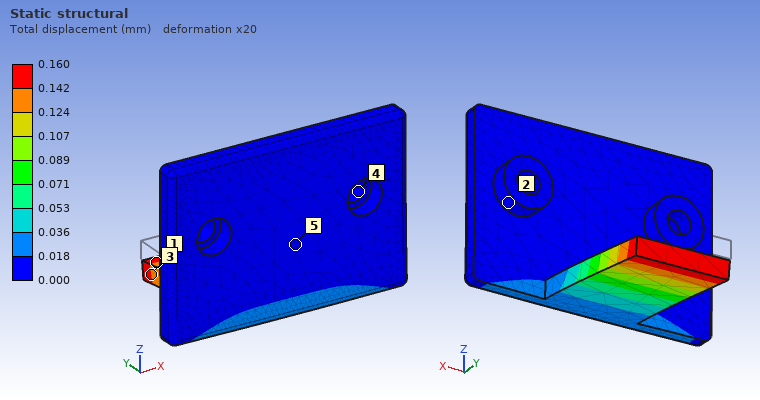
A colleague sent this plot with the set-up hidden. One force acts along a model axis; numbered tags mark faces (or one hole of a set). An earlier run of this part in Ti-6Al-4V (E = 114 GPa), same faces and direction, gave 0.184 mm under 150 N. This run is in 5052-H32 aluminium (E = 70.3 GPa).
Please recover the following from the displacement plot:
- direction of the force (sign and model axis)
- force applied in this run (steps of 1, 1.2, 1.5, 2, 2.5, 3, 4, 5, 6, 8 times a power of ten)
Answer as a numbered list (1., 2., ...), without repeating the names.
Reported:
1. -Z
2. 80 N
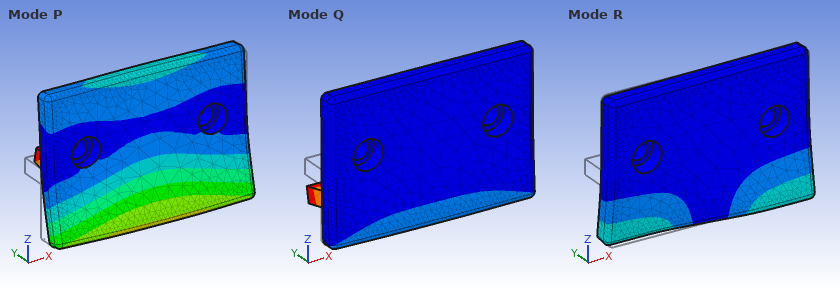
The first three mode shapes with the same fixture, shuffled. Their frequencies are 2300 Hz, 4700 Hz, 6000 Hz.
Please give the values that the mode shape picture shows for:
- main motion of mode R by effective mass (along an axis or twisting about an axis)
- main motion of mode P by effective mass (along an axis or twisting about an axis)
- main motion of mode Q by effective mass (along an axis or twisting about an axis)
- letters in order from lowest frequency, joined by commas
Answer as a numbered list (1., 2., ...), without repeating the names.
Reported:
1. along X
2. along Y
3. along Z
4. Q, R, P
